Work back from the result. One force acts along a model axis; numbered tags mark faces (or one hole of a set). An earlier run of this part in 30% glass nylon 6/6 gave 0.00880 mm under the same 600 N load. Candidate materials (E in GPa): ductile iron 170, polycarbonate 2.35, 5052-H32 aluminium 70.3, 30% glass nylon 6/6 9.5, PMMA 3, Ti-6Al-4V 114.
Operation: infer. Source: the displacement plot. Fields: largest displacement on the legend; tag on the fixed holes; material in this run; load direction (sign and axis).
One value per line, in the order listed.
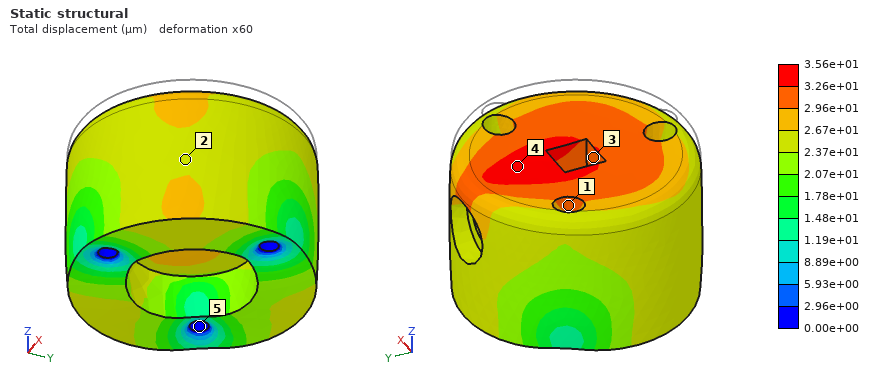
3.56e+01 µm
5
polycarbonate
-Z
